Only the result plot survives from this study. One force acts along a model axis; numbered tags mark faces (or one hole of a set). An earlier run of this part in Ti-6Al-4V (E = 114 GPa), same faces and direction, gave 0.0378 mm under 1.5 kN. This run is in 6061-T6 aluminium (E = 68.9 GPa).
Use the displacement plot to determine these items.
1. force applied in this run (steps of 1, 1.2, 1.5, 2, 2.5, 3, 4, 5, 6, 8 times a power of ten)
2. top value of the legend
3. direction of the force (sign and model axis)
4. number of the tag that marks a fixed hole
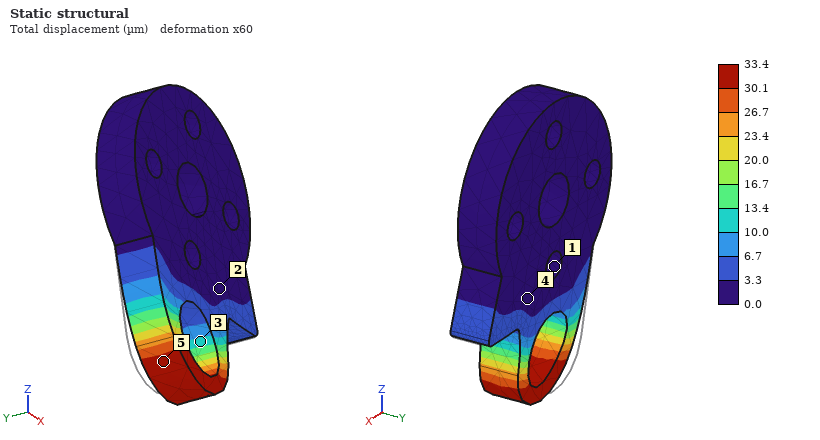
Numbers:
800 N
33.4 µm
+X
1
